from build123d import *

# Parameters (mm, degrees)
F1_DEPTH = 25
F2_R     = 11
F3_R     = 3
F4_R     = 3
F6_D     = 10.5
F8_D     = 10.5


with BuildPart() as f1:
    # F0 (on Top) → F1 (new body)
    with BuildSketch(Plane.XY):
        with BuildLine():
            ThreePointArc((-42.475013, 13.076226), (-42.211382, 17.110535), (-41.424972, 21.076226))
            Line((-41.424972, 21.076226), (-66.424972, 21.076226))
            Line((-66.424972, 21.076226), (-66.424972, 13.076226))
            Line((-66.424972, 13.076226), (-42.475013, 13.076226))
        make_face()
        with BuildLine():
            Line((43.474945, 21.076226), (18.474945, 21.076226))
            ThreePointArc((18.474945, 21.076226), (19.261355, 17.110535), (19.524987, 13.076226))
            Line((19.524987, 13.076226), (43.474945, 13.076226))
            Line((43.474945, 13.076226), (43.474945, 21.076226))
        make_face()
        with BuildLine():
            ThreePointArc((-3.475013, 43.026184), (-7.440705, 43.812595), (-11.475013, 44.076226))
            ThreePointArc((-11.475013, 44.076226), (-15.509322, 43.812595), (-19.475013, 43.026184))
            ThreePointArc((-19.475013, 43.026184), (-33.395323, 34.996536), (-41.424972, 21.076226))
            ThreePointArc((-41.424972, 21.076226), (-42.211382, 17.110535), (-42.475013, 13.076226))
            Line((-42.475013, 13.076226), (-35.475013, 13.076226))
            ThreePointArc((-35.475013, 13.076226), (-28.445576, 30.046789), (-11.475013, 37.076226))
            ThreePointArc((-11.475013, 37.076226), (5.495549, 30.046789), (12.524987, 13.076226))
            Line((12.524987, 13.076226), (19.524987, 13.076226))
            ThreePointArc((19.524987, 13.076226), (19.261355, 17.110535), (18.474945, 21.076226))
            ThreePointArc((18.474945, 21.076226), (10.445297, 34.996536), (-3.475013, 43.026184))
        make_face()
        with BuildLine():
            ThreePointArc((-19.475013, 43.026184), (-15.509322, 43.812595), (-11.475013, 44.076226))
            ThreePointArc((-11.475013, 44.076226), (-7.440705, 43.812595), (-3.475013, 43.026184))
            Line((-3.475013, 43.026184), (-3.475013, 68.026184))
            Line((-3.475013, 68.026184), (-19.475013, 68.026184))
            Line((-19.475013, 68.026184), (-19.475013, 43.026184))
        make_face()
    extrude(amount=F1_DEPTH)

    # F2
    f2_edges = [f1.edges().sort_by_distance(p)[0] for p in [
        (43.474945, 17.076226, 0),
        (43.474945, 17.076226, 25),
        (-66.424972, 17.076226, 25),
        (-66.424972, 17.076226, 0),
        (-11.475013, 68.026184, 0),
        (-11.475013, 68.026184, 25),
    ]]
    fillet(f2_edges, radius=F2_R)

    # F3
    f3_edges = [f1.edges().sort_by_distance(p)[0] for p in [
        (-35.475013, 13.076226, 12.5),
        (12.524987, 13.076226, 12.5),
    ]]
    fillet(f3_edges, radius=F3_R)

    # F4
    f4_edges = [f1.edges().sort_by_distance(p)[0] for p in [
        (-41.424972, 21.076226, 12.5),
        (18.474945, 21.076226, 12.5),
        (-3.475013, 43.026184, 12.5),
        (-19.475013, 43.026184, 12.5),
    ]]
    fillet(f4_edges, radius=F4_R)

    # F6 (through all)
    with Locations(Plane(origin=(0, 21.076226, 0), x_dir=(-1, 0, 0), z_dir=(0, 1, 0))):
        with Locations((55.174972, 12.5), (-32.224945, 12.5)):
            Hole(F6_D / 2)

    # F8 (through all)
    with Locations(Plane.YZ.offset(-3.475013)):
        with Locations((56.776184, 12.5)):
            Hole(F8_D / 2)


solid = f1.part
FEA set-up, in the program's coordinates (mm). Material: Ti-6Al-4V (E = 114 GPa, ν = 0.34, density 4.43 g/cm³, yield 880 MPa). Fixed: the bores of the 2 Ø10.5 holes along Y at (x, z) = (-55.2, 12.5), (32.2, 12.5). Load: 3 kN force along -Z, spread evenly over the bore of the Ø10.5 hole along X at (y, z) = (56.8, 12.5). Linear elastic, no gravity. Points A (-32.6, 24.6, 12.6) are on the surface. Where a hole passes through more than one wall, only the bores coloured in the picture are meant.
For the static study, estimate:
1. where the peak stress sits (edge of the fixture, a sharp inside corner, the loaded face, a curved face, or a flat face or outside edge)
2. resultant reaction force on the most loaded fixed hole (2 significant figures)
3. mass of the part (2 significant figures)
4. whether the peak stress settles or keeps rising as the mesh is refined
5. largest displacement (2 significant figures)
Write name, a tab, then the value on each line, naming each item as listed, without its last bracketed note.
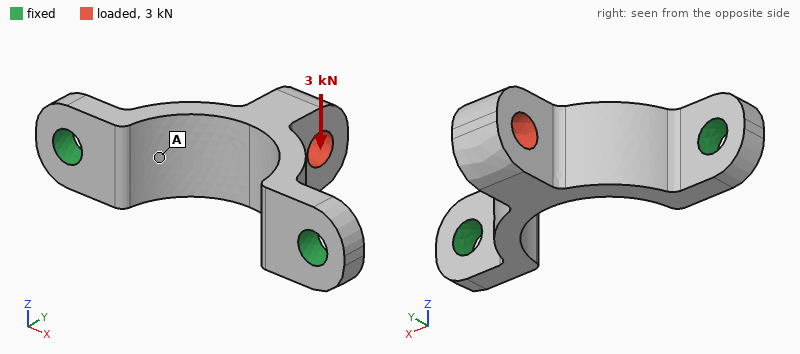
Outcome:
where the peak stress sits	edge of the fixture
resultant reaction force on the most loaded fixed hole	1.5 kN
mass of the part	130 g
whether the peak stress settles or keeps rising as the mesh is refined	keeps rising
largest displacement	0.31 mm
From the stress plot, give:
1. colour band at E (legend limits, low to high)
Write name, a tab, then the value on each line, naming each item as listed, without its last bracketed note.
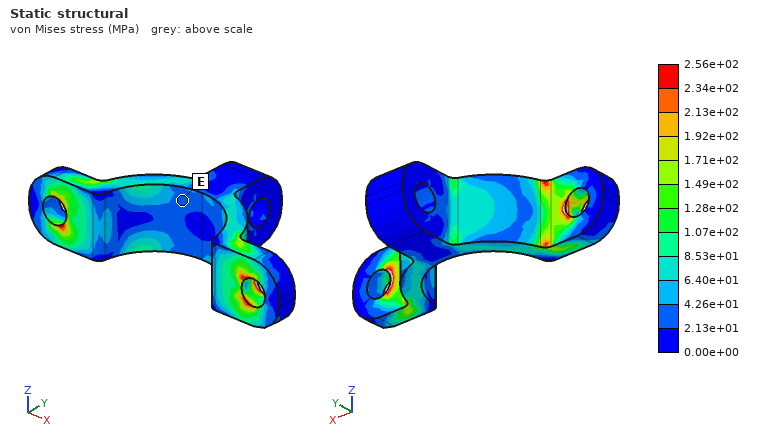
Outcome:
colour band at E	2.13e+01 to 4.26e+01 MPa
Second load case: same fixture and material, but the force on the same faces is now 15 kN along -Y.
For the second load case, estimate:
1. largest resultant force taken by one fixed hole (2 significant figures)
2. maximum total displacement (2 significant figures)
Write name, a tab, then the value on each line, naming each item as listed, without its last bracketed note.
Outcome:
largest resultant force taken by one fixed hole	11 kN
maximum total displacement	73 µm
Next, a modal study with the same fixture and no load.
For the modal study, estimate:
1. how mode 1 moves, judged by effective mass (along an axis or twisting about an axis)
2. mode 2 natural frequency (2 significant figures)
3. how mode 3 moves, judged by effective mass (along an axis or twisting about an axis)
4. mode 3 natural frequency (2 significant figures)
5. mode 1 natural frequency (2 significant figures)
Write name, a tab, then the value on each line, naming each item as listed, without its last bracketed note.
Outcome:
how mode 1 moves, judged by effective mass	along Z
mode 2 natural frequency	7400 Hz
how mode 3 moves, judged by effective mass	along Y
mode 3 natural frequency	9100 Hz
mode 1 natural frequency	2800 Hz
